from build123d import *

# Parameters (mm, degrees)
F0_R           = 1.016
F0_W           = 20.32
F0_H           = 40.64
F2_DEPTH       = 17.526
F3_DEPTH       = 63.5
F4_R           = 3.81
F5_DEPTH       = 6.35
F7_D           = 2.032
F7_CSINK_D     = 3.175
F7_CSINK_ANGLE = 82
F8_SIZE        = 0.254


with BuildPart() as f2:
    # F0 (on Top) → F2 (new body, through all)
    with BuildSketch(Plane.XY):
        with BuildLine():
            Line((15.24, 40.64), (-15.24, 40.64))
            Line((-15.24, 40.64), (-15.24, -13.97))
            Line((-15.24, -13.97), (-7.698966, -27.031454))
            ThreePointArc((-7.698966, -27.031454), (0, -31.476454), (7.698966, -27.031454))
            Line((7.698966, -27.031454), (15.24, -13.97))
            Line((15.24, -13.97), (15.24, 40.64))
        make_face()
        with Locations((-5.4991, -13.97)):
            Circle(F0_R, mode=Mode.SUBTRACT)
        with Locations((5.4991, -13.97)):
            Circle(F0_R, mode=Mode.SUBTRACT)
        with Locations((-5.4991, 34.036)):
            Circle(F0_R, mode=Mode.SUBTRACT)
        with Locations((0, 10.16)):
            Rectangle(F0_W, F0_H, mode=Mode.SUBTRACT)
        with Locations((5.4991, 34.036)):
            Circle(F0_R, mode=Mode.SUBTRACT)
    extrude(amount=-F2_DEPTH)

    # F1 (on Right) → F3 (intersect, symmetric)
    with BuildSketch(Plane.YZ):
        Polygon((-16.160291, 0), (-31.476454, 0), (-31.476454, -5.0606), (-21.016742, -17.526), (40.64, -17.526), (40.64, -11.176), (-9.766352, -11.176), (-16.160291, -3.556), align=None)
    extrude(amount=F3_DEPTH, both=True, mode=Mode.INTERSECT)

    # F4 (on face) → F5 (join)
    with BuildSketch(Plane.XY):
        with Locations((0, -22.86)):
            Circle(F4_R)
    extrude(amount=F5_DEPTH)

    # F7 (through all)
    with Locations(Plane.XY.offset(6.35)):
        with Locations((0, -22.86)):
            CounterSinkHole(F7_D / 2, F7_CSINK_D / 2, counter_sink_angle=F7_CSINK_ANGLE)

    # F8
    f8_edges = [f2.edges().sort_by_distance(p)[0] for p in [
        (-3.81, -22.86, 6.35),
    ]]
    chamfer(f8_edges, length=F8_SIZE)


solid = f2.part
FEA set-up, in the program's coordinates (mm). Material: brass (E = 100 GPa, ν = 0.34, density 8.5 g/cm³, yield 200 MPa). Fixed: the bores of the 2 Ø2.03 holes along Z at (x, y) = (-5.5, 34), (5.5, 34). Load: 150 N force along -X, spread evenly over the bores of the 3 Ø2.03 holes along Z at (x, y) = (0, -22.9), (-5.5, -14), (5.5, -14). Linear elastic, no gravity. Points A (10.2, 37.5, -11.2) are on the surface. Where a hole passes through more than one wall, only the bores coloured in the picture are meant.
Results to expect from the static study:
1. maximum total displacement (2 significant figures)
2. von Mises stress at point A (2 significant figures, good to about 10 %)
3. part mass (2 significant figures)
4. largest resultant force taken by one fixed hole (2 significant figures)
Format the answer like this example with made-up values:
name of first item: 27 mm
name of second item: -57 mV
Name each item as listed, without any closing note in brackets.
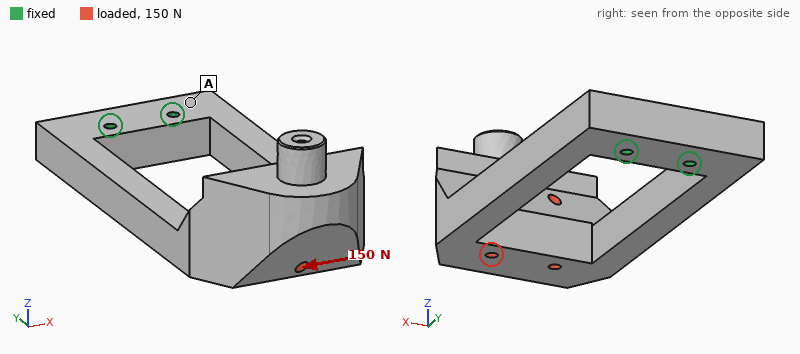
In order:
maximum total displacement: 0.15 mm
von Mises stress at point A: 12 MPa
part mass: 91 g
largest resultant force taken by one fixed hole: 560 N
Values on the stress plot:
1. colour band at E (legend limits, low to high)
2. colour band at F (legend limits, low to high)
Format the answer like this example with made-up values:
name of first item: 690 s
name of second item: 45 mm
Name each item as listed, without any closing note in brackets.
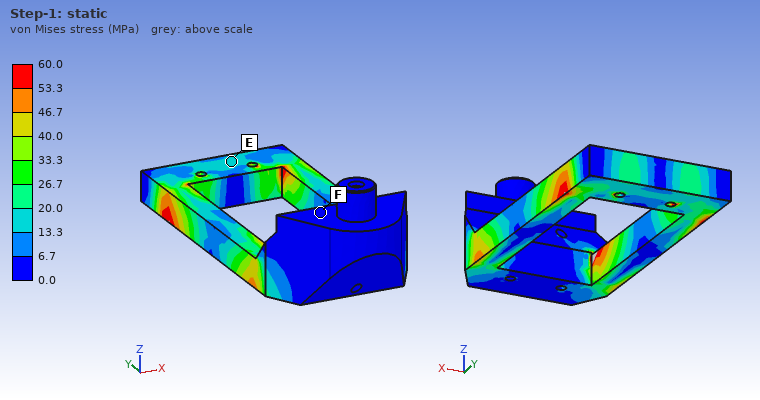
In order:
colour band at E: 13.3 to 20.0 MPa
colour band at F: 0.0 to 6.7 MPa
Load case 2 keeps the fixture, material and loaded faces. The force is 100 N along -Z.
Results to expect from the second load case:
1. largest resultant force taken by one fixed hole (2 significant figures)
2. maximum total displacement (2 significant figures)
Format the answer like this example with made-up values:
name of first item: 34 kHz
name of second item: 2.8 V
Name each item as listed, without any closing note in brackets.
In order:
largest resultant force taken by one fixed hole: 50 N
maximum total displacement: 0.37 mm
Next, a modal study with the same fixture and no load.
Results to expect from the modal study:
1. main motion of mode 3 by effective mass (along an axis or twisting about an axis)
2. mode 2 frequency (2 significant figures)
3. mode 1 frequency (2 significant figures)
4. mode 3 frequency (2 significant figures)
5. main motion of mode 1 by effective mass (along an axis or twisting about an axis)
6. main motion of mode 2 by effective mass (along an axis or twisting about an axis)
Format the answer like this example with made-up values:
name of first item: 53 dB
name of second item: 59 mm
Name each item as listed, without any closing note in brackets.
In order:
main motion of mode 3 by effective mass: twisting about Y
mode 2 frequency: 710 Hz
mode 1 frequency: 390 Hz
mode 3 frequency: 1600 Hz
main motion of mode 1 by effective mass: along Z
main motion of mode 2 by effective mass: along X
